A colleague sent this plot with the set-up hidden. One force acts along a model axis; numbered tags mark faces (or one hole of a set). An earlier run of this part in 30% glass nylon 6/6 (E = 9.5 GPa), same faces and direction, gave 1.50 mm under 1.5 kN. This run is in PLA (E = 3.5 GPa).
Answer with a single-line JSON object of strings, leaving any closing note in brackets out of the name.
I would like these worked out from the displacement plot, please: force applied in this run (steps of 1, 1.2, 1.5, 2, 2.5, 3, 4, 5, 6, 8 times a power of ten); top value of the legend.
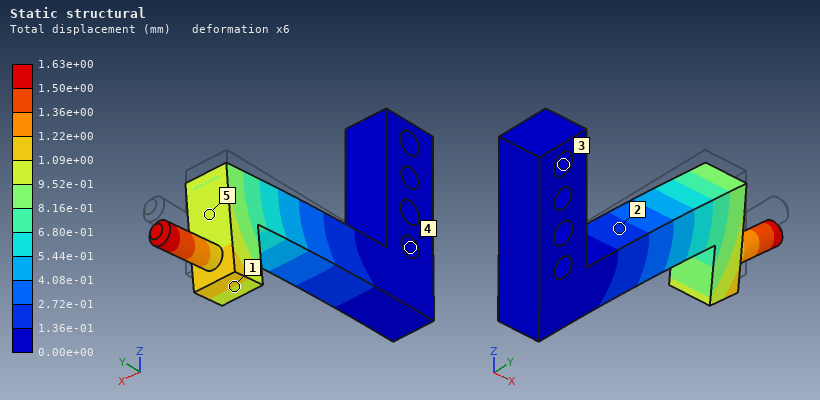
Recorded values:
{"force applied in this run": "600 N", "top value of the legend": "1.63e+00 mm"}
